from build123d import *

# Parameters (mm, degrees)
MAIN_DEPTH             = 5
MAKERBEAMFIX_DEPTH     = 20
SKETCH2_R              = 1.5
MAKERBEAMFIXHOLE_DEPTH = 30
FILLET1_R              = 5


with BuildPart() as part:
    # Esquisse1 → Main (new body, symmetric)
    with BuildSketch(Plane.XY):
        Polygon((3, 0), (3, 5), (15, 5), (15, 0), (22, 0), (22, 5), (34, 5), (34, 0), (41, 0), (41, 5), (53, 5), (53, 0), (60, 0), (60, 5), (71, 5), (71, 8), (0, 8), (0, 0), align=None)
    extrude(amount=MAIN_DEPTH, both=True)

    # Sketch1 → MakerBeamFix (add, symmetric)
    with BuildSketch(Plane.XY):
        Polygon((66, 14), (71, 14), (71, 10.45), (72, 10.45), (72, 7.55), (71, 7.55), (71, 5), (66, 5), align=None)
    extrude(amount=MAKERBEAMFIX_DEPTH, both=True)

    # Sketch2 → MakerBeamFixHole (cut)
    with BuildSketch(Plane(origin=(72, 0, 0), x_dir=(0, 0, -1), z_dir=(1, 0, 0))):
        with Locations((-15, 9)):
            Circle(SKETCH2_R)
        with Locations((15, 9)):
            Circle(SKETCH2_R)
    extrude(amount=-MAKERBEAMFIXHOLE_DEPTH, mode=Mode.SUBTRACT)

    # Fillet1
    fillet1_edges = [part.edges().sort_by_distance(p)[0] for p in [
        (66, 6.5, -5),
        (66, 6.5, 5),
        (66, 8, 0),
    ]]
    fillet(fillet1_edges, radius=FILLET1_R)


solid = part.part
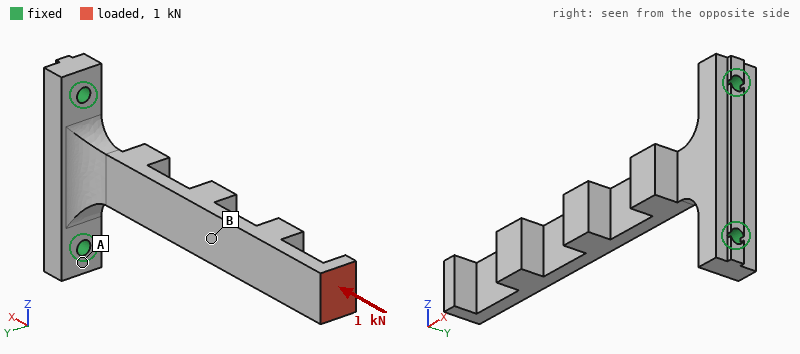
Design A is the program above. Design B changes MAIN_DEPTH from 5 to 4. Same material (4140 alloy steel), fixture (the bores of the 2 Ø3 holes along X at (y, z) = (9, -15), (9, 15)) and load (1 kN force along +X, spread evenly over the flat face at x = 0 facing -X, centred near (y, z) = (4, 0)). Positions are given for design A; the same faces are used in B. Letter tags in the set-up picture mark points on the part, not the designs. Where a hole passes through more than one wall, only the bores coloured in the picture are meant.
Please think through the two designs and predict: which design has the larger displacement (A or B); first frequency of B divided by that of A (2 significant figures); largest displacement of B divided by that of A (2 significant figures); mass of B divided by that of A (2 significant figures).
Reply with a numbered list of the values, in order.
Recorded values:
1. B
2. 1.0
3. 1.2
4. 0.87
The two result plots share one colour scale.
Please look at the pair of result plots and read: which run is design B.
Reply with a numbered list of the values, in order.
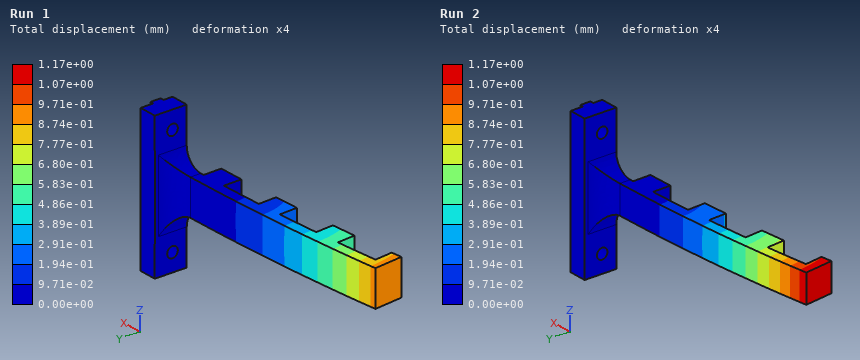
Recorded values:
1. Run 2
